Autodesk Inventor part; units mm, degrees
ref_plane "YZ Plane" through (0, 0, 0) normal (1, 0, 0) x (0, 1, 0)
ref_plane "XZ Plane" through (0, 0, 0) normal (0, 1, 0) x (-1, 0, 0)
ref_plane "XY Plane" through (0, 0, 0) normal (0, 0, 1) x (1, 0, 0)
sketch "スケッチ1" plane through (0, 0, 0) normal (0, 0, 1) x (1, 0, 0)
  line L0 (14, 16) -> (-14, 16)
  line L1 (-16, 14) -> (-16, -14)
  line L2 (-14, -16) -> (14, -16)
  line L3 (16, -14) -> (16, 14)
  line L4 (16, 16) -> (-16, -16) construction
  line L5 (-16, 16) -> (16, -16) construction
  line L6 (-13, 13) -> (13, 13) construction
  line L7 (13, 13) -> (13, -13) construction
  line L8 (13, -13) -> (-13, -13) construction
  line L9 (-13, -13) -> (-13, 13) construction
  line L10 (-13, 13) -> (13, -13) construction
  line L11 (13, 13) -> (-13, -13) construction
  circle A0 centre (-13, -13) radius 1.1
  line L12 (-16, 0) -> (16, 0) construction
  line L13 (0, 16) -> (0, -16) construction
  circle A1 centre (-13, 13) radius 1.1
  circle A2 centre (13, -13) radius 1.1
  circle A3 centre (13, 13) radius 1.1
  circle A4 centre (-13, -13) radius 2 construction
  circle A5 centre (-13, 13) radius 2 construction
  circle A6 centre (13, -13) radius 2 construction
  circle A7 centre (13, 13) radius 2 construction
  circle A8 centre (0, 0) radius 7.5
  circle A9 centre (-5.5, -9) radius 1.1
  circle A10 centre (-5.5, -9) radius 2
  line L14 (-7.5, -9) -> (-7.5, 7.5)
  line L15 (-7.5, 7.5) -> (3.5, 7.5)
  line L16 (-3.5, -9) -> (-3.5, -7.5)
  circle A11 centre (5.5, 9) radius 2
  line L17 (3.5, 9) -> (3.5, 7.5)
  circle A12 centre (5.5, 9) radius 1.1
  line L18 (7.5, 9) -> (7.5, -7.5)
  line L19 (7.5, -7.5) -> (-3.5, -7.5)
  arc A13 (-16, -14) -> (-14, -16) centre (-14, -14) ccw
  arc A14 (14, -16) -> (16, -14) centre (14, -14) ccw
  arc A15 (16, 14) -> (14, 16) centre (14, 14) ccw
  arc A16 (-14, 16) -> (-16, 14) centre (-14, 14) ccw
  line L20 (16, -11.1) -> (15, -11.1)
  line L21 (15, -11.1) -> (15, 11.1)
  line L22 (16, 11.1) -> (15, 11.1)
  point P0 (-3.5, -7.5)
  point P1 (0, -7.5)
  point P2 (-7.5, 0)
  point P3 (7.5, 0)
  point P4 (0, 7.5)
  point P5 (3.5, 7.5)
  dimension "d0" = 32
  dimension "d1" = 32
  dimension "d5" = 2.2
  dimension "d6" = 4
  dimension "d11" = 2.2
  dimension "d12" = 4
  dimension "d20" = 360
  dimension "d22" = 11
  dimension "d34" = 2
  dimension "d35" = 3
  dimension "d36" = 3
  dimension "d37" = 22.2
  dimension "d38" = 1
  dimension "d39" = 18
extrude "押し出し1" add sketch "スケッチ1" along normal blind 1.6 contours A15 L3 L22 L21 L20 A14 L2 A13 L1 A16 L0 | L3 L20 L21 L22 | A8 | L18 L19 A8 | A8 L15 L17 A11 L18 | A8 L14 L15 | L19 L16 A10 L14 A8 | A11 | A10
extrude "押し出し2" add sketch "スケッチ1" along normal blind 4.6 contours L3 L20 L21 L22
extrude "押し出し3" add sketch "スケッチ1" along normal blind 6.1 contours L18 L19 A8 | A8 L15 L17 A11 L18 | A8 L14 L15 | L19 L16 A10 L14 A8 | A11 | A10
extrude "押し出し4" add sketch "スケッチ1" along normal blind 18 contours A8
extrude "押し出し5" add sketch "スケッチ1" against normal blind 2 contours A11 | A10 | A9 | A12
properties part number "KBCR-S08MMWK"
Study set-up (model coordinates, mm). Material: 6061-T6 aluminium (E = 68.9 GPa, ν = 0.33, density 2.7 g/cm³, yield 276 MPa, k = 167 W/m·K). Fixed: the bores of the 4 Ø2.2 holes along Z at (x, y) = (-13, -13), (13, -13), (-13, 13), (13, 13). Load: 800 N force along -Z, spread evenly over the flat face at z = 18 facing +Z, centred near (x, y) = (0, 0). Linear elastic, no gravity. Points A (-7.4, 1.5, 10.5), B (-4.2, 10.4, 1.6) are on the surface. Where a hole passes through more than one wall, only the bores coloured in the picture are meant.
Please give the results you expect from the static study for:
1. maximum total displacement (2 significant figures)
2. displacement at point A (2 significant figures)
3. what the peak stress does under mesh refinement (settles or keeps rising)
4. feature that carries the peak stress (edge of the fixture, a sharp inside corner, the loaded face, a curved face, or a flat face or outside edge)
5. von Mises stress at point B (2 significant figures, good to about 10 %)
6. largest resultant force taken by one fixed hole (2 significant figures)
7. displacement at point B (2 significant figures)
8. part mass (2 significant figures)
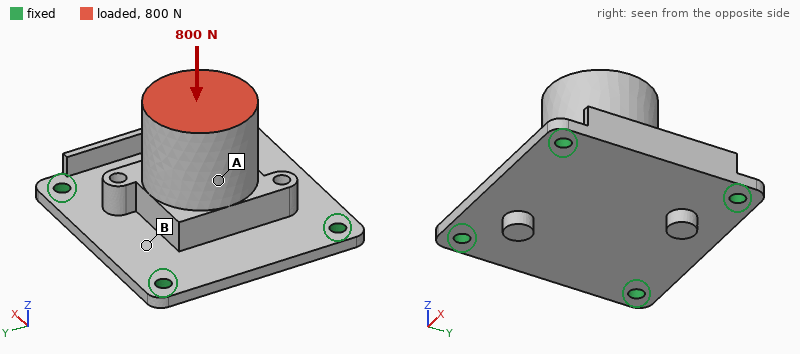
50 µm
49 µm
keeps rising
edge of the fixture
48 MPa
260 N
41 µm
13 g
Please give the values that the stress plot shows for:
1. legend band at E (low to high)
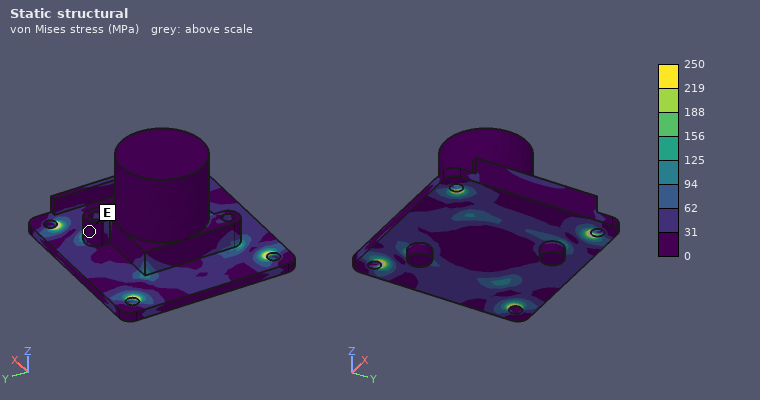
0 to 31 MPa
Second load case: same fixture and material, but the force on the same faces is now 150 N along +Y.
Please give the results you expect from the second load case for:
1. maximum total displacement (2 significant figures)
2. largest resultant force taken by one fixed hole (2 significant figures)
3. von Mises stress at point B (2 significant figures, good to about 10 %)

27 µm
72 N
21 MPa
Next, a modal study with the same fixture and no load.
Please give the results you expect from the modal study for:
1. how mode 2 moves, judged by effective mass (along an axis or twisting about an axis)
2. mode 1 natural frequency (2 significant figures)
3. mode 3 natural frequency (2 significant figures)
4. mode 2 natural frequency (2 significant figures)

along Z
6000 Hz
7200 Hz
6300 Hz
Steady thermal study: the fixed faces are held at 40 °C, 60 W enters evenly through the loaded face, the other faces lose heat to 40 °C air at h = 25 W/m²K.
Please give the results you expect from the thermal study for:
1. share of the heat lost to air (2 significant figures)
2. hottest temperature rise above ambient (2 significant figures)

5.1 %
80 K
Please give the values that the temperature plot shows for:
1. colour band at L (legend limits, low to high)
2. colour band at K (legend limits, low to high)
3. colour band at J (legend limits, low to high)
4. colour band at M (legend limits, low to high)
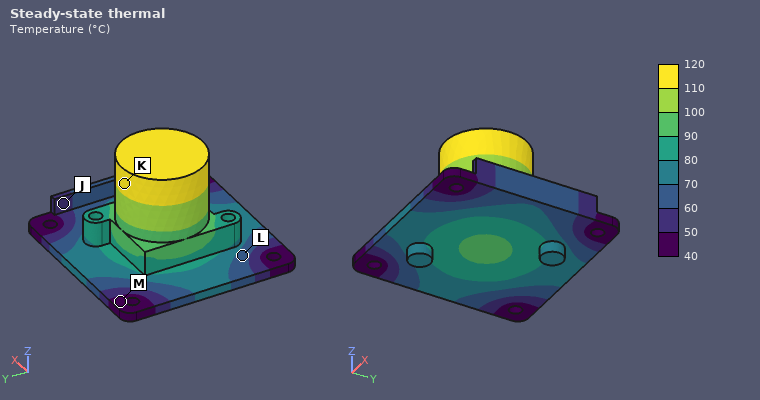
60 to 70 °C
110 to 120 °C
50 to 60 °C
40 to 50 °C
